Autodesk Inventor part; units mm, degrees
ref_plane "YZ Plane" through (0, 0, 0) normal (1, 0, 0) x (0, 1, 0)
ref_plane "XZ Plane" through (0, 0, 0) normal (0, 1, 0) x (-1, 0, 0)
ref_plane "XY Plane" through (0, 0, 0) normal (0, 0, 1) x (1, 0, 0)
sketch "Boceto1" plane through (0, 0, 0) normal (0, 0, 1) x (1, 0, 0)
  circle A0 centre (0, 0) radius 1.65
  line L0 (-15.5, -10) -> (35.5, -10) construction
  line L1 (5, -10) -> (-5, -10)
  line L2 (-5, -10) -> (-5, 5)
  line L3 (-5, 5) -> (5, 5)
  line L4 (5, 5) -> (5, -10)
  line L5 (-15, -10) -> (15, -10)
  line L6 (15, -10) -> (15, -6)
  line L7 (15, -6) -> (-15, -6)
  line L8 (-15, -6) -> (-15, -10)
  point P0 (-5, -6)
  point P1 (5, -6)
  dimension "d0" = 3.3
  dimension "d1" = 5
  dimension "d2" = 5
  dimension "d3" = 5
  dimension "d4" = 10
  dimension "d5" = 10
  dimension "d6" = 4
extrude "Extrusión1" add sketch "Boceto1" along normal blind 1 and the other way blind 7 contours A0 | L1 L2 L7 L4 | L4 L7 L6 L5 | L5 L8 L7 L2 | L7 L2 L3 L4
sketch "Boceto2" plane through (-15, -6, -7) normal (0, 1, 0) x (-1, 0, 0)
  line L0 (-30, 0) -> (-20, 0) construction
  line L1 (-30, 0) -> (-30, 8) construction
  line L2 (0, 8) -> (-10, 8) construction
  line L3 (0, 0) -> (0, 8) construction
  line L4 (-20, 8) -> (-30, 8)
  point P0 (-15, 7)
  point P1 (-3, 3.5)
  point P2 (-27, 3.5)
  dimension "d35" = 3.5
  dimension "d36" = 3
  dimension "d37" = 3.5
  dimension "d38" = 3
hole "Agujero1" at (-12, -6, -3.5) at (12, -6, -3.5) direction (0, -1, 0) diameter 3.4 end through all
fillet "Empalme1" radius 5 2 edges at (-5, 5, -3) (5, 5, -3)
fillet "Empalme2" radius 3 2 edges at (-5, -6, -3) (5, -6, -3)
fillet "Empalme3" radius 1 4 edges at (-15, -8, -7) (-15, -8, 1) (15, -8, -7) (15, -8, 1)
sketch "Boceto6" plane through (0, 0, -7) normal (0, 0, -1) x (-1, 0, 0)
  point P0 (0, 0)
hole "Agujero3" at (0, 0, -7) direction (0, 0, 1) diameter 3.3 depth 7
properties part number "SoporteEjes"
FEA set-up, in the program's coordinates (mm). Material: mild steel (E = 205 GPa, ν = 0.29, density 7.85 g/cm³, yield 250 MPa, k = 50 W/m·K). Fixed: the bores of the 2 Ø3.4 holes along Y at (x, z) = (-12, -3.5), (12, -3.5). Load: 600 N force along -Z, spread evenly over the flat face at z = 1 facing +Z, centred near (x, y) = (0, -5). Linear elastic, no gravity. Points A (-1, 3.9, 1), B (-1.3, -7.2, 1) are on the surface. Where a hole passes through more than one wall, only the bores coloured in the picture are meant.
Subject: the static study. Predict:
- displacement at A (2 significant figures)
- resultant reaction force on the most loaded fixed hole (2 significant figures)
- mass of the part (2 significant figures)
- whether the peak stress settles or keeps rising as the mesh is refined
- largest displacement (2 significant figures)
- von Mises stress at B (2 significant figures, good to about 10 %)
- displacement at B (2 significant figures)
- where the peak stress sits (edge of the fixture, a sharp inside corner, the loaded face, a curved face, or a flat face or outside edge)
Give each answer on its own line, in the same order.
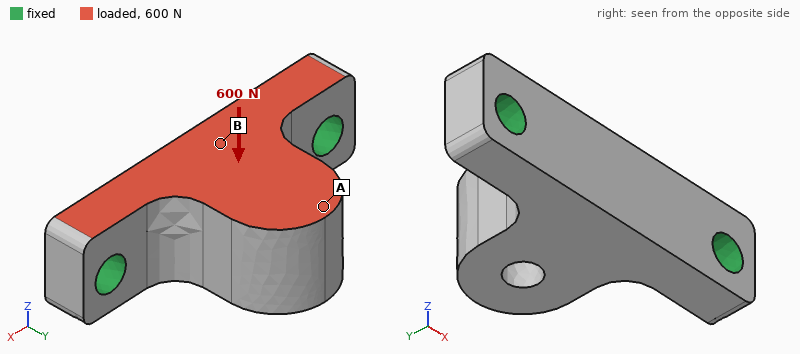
9.3 µm
300 N
13 g
keeps rising
10.0 µm
16 MPa
3.1 µm
edge of the fixture
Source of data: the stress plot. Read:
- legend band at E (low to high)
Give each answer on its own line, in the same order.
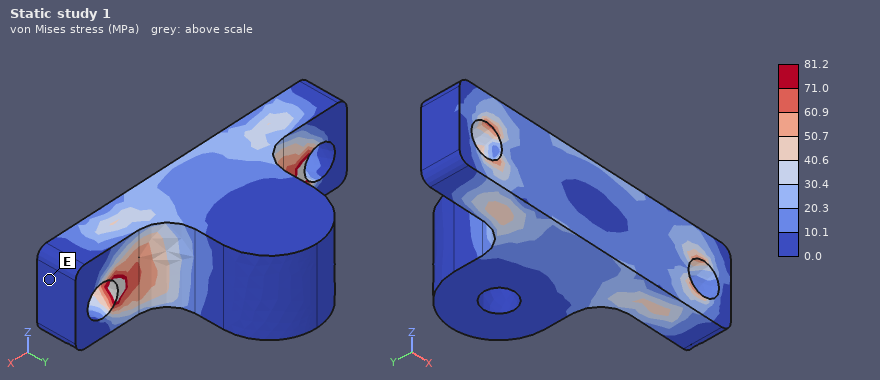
0.0 to 10.1 MPa
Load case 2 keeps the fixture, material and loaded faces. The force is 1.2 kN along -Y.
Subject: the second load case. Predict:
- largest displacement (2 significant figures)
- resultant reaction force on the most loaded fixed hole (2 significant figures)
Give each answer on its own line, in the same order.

18 µm
630 N
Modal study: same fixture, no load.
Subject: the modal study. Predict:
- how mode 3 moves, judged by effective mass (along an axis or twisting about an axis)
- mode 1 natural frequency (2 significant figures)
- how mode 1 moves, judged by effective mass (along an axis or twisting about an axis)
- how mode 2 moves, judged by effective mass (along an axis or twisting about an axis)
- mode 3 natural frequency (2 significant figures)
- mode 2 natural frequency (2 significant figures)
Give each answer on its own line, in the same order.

along X
14 kHz
along Z
along Y
33 kHz
29 kHz
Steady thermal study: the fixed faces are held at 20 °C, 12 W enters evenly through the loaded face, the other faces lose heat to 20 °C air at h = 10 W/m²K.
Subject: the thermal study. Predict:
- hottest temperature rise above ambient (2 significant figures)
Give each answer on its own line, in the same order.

32 K
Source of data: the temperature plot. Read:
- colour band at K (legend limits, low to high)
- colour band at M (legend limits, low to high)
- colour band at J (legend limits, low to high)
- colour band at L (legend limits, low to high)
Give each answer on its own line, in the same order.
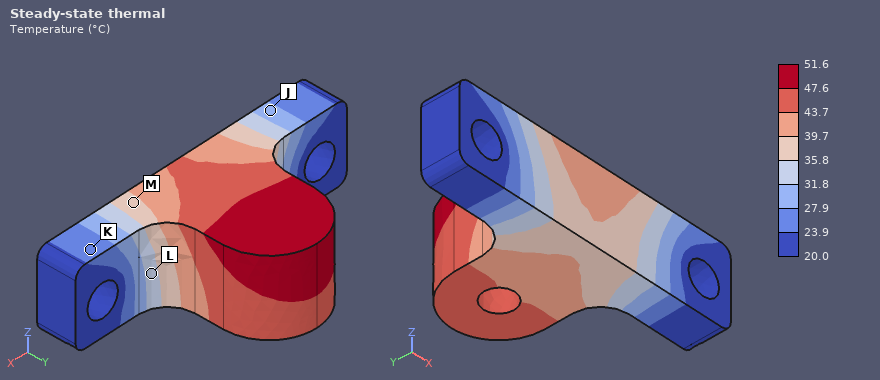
23.9 to 27.9 °C
35.8 to 39.7 °C
27.9 to 31.8 °C
31.8 to 35.8 °C
